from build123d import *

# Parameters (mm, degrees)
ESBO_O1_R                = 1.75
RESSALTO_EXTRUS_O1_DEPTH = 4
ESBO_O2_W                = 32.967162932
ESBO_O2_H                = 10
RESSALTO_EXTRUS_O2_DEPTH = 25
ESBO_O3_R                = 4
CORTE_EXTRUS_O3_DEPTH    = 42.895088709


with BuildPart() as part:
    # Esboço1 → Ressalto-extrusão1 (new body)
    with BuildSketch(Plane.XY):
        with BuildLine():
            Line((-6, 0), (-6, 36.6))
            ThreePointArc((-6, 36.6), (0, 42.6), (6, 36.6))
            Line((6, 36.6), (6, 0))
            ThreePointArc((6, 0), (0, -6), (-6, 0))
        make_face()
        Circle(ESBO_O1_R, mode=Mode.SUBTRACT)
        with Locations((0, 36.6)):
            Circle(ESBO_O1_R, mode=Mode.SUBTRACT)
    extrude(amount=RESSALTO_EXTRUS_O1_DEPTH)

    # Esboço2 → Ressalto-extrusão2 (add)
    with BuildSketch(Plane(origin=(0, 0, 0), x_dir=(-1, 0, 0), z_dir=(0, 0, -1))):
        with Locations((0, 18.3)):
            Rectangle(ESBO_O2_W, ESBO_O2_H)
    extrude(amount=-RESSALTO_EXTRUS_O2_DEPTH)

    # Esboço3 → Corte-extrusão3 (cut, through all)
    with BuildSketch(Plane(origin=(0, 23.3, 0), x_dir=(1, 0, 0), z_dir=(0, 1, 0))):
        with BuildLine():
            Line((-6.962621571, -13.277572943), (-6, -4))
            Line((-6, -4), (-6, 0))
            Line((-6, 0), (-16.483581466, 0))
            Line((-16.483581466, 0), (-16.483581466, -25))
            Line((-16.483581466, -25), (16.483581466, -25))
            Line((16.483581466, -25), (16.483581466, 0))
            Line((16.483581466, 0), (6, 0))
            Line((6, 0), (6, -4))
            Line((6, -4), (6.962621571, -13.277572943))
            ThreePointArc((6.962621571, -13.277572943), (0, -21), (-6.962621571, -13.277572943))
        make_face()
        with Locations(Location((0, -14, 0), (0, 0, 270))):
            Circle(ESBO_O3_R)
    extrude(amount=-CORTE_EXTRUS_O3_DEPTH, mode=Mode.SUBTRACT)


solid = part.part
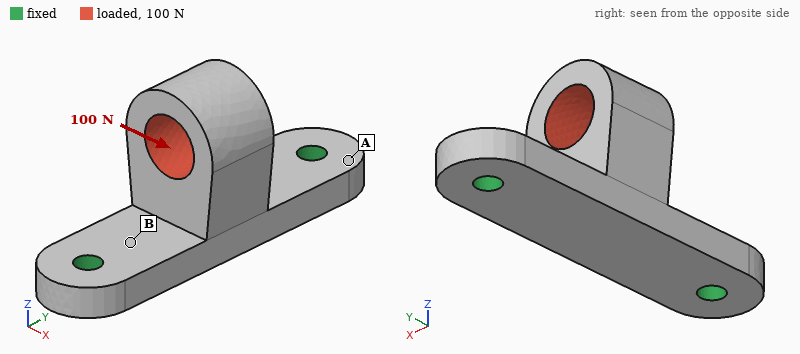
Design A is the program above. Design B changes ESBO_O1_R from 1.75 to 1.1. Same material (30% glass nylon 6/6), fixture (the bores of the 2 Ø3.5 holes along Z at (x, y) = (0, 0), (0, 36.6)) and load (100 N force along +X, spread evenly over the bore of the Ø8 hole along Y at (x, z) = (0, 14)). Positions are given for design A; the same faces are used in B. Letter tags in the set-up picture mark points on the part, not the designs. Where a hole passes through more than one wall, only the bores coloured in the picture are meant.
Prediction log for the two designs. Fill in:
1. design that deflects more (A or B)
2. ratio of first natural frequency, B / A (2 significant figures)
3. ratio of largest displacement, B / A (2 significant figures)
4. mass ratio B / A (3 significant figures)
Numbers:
B
0.94
1.1
1.01
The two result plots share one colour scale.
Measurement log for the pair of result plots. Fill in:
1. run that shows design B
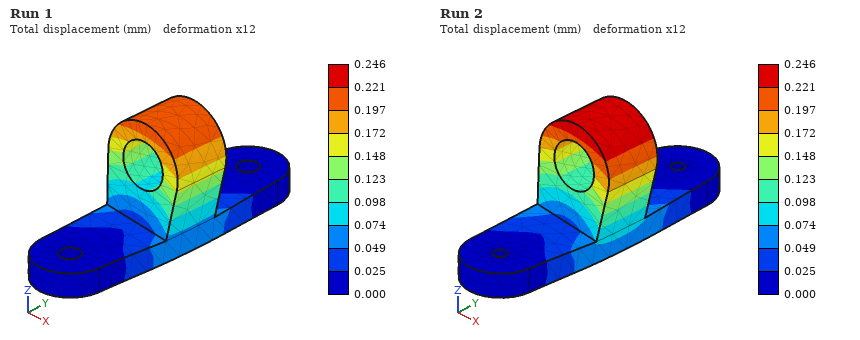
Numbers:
Run 2
